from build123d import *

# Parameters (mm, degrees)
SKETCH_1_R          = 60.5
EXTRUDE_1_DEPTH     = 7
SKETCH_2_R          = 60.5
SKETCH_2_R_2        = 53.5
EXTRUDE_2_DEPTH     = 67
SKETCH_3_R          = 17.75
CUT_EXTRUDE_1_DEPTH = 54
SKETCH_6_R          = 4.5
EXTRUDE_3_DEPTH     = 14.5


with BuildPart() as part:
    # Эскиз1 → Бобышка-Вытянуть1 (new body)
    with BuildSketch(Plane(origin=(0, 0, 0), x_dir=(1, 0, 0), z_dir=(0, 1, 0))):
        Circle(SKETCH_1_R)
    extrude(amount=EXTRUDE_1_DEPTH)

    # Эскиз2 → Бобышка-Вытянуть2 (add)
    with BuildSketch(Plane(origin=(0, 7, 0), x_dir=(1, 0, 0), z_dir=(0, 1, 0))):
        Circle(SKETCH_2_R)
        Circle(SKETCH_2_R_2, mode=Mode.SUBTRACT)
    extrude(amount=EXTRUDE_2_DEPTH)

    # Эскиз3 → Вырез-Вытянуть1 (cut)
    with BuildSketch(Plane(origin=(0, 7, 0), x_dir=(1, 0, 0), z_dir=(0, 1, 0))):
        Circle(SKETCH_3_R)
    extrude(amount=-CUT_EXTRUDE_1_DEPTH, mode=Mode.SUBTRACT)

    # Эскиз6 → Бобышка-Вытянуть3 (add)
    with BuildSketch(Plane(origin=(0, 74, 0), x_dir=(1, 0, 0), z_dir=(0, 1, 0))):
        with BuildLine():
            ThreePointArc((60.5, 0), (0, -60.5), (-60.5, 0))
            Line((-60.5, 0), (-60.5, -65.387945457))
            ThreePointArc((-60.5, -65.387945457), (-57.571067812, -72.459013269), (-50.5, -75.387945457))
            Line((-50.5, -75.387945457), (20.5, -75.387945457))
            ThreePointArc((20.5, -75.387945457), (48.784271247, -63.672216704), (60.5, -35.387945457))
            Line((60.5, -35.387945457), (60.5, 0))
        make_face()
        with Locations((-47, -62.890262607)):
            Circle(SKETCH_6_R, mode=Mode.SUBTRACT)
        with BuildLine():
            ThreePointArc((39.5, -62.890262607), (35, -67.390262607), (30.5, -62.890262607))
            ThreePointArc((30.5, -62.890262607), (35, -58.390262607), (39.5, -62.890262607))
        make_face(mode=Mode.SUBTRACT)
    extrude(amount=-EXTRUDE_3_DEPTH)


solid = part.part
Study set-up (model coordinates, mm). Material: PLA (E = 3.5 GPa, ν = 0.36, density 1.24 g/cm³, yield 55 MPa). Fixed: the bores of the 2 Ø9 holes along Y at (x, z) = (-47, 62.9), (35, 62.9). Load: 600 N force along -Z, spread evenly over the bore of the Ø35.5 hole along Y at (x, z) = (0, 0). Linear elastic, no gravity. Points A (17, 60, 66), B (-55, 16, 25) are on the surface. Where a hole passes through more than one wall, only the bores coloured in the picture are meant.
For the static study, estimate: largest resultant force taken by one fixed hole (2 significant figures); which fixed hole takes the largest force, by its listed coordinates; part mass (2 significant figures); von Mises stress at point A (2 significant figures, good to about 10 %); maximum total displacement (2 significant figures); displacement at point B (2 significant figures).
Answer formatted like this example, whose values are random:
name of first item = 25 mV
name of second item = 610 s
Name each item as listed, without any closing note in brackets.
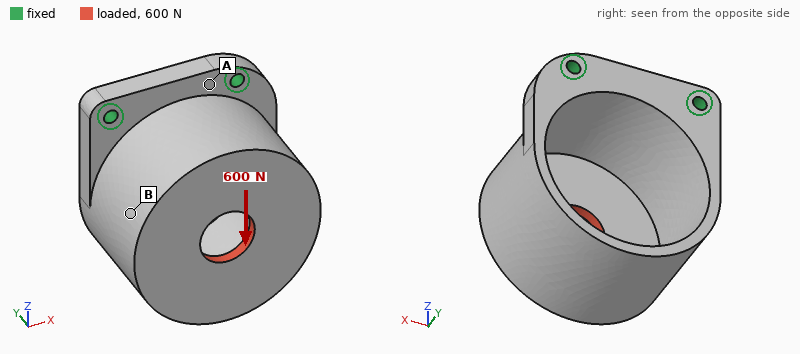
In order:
largest resultant force taken by one fixed hole = 380 N
which fixed hole takes the largest force, by its listed coordinates = (35, 62.9)
part mass = 350 g
von Mises stress at point A = 4.2 MPa
maximum total displacement = 2.0 mm
displacement at point B = 0.84 mm
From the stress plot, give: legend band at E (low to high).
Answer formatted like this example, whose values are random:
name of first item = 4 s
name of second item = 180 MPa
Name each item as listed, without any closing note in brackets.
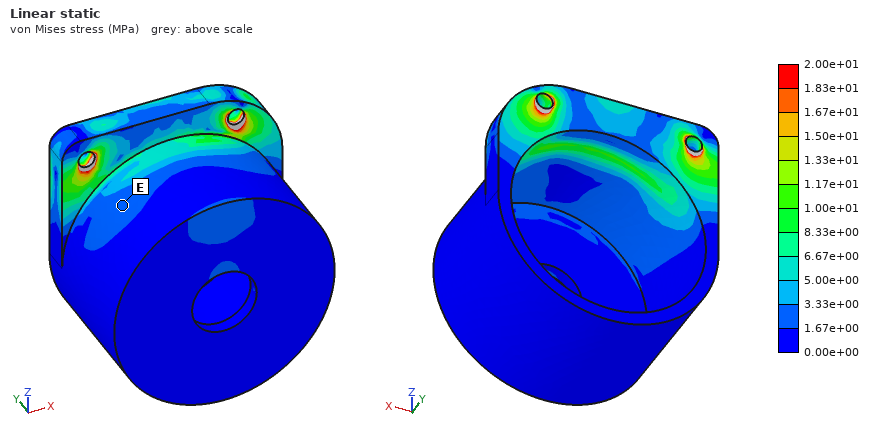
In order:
legend band at E = 1.67e+00 to 3.33e+00 MPa
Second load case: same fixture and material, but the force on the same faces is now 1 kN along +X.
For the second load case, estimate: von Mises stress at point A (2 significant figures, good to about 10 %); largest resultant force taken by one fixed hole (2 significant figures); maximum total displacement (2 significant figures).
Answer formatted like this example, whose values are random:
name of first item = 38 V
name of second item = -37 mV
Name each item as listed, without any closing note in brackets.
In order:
von Mises stress at point A = 3.5 MPa
largest resultant force taken by one fixed hole = 1.1 kN
maximum total displacement = 1.2 mm
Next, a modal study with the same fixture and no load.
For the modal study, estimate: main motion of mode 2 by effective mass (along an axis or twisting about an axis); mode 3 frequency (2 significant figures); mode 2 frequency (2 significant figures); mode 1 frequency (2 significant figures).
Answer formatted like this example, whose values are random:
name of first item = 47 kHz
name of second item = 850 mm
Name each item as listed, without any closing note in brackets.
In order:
main motion of mode 2 by effective mass = along X
mode 3 frequency = 750 Hz
mode 2 frequency = 290 Hz
mode 1 frequency = 190 Hz
